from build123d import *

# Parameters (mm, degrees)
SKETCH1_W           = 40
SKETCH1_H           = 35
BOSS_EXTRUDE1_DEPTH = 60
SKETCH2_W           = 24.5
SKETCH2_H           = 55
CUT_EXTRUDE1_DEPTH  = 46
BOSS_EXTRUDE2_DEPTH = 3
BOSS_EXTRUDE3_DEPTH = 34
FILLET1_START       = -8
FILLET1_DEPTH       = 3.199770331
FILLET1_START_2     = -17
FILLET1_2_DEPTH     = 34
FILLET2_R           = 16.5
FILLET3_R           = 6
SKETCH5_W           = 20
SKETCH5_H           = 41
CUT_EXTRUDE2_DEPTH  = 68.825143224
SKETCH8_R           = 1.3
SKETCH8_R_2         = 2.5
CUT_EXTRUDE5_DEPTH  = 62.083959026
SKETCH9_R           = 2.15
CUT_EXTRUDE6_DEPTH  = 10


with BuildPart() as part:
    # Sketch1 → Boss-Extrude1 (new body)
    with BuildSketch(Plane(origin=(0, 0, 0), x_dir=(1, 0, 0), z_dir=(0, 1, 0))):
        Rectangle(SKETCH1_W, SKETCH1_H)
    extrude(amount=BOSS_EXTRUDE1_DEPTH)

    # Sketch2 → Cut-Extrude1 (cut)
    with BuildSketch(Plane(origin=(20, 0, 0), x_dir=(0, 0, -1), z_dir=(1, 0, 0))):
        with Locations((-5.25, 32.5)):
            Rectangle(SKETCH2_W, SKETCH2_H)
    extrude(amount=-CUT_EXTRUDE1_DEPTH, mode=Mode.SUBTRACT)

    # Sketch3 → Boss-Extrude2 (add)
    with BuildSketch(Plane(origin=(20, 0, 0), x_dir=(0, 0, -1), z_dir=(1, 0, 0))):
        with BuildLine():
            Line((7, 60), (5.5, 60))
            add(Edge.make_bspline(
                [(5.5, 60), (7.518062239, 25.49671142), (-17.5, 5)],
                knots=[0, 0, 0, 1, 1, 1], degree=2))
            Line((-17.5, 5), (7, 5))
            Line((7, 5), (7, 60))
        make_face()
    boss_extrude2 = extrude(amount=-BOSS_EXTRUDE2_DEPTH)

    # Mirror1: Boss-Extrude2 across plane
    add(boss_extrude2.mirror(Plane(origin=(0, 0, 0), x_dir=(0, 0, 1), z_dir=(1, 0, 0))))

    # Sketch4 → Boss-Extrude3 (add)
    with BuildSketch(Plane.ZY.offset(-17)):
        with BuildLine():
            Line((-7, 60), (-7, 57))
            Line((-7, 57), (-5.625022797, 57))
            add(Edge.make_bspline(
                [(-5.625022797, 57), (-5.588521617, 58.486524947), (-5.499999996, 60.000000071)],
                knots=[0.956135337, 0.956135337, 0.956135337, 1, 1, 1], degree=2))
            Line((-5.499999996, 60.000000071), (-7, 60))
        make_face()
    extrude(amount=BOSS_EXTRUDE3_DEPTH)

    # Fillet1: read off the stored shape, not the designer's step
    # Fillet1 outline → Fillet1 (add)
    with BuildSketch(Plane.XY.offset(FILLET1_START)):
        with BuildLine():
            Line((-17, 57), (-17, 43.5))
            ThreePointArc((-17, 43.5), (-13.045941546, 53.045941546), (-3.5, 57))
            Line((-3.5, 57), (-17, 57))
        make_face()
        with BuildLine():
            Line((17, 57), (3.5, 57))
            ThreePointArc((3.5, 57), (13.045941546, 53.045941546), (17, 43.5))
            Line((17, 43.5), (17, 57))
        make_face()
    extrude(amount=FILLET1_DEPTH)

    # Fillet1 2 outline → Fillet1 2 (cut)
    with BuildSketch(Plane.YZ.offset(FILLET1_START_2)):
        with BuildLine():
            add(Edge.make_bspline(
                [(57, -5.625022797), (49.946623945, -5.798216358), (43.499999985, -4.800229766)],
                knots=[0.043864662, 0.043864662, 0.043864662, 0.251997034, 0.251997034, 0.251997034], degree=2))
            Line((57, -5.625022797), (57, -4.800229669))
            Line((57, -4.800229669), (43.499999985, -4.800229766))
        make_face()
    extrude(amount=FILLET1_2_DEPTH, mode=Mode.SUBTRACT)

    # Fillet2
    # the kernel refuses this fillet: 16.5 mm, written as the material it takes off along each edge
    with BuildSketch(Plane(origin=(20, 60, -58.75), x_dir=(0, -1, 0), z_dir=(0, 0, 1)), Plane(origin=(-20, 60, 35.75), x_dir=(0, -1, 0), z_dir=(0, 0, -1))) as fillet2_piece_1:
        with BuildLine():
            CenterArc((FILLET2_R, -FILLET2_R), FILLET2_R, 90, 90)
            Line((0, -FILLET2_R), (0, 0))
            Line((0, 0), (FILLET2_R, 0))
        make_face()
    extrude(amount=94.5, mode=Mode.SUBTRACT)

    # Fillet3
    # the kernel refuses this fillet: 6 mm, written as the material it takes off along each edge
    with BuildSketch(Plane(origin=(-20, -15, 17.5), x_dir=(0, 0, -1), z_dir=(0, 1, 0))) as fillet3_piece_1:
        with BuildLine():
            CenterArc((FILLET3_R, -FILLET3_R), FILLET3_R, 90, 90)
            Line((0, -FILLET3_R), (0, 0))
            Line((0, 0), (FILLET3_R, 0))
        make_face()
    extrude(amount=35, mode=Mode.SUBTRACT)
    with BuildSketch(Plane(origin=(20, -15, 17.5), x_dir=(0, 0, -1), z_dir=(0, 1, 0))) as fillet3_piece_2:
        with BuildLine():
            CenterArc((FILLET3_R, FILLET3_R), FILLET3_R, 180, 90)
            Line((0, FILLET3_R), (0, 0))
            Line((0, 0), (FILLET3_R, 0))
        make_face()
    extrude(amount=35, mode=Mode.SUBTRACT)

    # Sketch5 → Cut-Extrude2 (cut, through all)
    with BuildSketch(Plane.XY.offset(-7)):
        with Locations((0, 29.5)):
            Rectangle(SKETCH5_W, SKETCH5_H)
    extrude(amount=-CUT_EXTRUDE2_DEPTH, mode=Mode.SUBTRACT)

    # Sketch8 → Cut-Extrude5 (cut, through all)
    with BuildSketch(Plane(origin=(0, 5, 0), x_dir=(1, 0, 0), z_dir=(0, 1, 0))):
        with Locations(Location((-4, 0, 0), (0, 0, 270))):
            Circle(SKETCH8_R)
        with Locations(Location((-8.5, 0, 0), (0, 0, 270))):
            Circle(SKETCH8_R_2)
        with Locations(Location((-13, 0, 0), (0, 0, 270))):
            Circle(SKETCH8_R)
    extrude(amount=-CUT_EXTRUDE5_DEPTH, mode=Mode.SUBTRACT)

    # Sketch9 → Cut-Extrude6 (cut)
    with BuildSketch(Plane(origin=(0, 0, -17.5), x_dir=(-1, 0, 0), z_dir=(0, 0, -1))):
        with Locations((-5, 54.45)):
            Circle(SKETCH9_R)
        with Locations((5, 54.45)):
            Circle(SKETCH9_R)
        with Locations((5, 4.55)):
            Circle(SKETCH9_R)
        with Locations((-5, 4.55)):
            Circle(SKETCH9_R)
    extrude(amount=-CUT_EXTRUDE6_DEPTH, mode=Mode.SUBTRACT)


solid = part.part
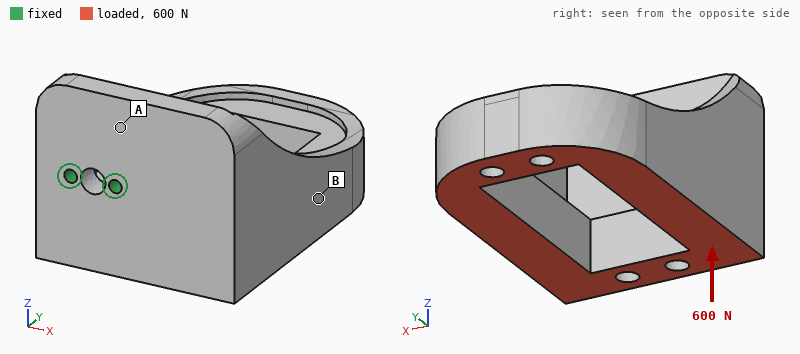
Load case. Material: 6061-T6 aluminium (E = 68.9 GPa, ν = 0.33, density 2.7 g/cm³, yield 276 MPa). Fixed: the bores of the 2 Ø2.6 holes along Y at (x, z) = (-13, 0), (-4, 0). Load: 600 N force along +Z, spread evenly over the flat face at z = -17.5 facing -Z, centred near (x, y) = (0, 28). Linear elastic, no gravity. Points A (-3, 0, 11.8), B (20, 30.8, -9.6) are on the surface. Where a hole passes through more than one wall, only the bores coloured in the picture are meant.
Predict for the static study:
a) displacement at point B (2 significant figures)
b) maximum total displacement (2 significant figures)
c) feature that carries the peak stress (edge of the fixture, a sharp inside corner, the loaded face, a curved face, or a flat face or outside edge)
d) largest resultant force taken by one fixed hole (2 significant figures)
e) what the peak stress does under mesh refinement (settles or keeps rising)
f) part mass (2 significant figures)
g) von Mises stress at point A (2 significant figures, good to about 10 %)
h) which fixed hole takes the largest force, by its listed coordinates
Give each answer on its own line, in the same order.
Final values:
0.13 mm
0.24 mm
edge of the fixture
750 N
keeps rising
59 g
29 MPa
(-4, 0)
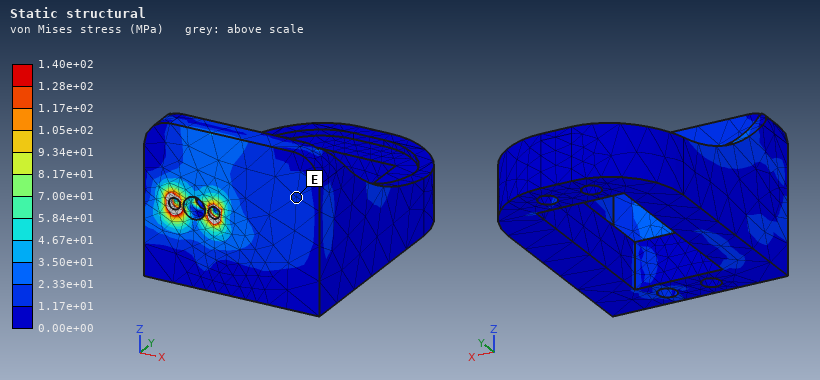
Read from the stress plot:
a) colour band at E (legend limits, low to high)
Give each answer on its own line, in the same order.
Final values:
1.17e+01 to 2.33e+01 MPa
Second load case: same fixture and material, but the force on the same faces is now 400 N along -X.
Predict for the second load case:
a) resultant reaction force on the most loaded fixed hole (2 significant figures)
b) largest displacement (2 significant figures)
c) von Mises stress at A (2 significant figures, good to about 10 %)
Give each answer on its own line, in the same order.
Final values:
910 N
100 µm
15 MPa
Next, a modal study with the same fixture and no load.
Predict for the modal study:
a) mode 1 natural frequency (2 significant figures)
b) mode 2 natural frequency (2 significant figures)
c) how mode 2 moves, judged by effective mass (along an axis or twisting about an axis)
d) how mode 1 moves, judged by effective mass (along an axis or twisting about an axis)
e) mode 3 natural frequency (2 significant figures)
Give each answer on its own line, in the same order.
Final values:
1400 Hz
1600 Hz
along X
along Z
4200 Hz
